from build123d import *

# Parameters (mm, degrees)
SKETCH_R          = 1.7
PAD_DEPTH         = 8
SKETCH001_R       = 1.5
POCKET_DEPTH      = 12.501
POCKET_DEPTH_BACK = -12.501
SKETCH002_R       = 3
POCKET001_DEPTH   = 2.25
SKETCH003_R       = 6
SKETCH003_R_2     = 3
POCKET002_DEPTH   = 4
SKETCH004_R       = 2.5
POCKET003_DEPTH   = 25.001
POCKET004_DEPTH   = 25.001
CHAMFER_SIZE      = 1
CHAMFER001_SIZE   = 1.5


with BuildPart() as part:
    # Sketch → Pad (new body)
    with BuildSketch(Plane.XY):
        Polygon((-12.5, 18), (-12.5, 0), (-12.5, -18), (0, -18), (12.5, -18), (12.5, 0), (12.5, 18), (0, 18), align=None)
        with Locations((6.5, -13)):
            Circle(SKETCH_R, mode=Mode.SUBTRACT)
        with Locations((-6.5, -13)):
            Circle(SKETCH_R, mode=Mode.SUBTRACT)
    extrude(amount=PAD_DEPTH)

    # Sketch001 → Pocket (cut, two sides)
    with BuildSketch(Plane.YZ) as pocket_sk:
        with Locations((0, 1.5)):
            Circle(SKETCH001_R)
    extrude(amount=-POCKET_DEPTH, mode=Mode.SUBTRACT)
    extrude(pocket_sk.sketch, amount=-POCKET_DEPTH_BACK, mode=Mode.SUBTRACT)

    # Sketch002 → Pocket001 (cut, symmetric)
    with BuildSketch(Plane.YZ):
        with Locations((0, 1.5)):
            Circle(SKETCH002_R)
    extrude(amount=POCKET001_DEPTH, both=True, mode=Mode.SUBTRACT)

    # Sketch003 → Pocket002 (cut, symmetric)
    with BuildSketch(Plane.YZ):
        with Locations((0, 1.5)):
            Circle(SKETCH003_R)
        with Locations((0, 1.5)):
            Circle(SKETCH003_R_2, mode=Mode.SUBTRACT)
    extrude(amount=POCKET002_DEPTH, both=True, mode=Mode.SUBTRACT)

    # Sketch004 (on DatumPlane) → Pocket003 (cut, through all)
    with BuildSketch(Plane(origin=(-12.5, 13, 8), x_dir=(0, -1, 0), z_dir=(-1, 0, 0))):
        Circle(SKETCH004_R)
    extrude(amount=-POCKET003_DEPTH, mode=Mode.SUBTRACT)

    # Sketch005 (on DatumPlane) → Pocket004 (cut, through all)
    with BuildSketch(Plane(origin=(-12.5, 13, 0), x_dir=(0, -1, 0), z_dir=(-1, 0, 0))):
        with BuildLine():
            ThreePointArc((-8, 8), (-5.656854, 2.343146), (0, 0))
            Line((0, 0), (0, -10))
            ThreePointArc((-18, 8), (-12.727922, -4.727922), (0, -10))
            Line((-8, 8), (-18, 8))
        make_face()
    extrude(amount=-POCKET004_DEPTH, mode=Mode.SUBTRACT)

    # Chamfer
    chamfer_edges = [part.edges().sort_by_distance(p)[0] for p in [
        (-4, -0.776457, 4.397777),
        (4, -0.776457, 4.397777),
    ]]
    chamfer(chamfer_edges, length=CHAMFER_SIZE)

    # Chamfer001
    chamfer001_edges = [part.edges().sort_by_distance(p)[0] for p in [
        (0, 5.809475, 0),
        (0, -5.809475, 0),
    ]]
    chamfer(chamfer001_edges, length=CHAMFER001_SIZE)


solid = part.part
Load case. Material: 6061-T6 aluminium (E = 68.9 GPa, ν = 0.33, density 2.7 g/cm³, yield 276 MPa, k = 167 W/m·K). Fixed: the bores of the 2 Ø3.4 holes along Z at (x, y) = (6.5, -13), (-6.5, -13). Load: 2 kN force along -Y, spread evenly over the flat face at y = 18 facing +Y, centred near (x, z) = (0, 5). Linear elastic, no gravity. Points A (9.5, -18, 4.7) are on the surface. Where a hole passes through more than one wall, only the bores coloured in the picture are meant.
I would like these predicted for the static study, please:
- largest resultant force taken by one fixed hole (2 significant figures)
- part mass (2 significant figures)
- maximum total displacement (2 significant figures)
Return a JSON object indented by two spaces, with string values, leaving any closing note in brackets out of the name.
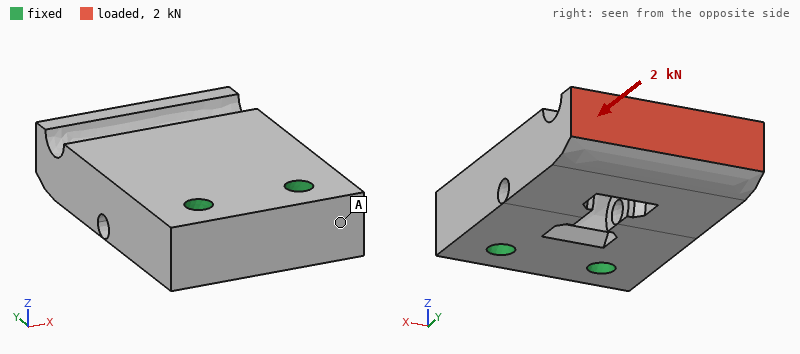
{
  "largest resultant force taken by one fixed hole": "1.0 kN",
  "part mass": "16 g",
  "maximum total displacement": "15 µm"
}
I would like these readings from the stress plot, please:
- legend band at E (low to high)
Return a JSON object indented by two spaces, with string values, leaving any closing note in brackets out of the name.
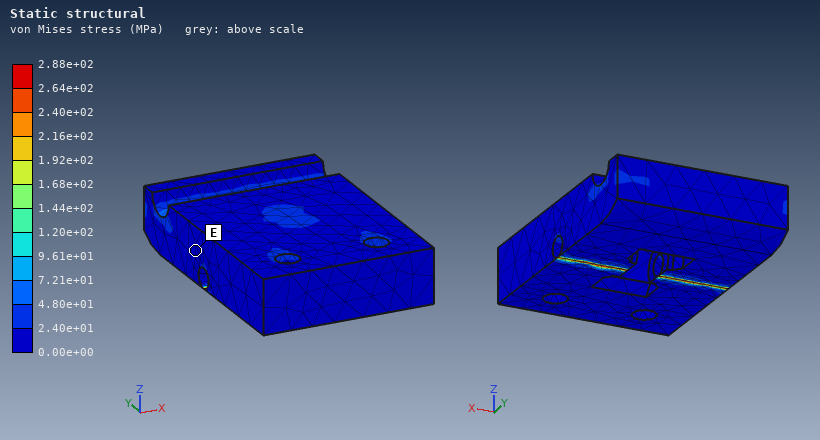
{
  "legend band at E": "0.00e+00 to 2.40e+01 MPa"
}
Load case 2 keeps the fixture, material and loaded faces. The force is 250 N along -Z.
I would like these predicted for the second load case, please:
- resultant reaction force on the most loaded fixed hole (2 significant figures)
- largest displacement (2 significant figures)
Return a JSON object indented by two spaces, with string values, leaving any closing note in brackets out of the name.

{
  "resultant reaction force on the most loaded fixed hole": "130 N",
  "largest displacement": "62 µm"
}
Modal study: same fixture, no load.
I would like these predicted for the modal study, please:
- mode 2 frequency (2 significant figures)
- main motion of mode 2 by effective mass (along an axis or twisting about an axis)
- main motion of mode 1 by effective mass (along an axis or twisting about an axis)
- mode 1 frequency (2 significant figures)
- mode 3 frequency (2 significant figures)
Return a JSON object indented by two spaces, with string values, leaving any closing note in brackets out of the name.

{
  "mode 2 frequency": "11 kHz",
  "main motion of mode 2 by effective mass": "along X",
  "main motion of mode 1 by effective mass": "along Z",
  "mode 1 frequency": "5700 Hz",
  "mode 3 frequency": "14 kHz"
}
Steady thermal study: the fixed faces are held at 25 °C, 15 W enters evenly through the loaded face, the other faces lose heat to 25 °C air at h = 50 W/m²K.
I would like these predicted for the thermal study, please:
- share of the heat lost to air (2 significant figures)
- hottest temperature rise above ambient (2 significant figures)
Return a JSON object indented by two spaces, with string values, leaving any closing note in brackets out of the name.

{
  "share of the heat lost to air": "7.4 %",
  "hottest temperature rise above ambient": "19 K"
}
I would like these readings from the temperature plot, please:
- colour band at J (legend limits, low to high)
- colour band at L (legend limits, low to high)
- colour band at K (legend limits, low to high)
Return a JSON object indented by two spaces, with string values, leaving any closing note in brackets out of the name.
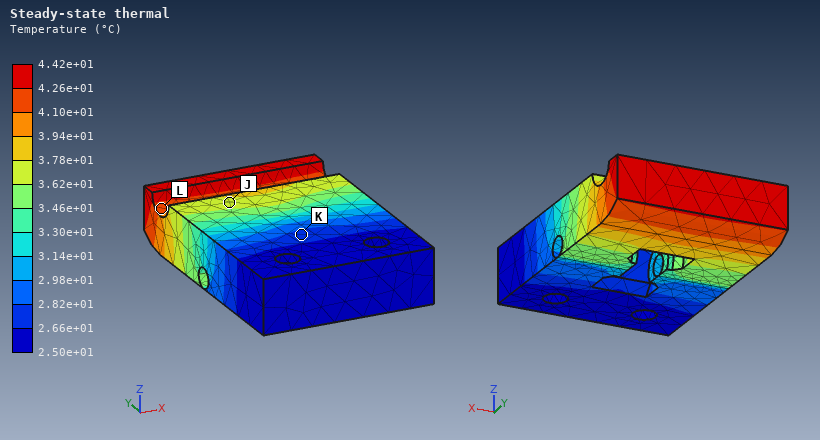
{
  "colour band at J": "3.62e+01 to 3.78e+01 °C",
  "colour band at L": "4.10e+01 to 4.26e+01 °C",
  "colour band at K": "2.66e+01 to 2.82e+01 °C"
}
